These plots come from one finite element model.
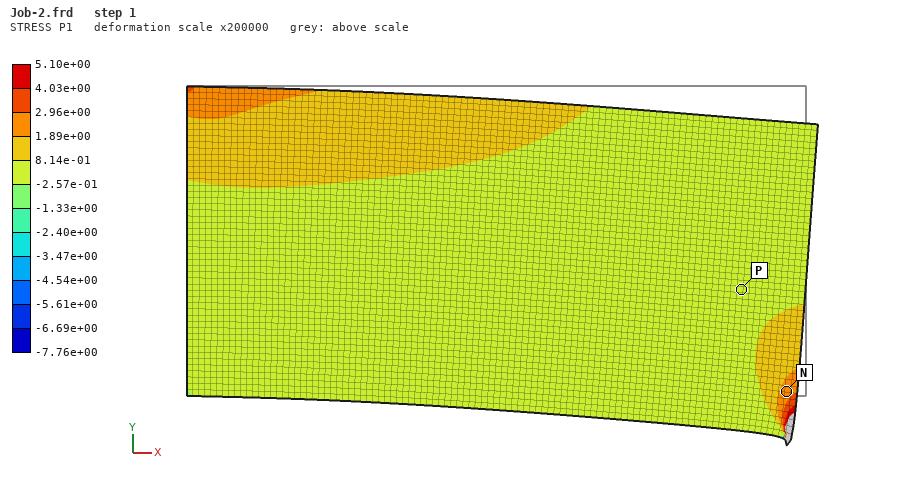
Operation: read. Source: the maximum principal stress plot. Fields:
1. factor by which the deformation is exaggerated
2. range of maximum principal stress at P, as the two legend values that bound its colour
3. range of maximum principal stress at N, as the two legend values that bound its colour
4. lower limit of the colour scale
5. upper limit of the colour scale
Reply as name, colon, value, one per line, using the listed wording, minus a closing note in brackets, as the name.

factor by which the deformation is exaggerated: 200000
range of maximum principal stress at P, as the two legend values that bound its colour: -2.57e-01 to 8.14e-01
range of maximum principal stress at N, as the two legend values that bound its colour: 1.89e+00 to 2.96e+00
lower limit of the colour scale: -7.76e+00
upper limit of the colour scale: 5.10e+00
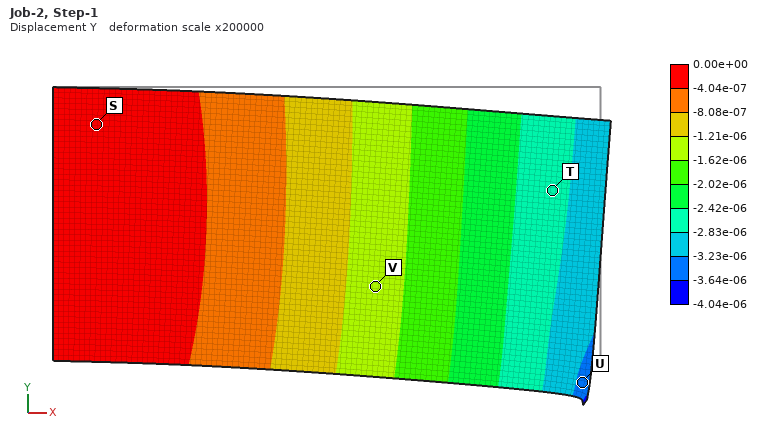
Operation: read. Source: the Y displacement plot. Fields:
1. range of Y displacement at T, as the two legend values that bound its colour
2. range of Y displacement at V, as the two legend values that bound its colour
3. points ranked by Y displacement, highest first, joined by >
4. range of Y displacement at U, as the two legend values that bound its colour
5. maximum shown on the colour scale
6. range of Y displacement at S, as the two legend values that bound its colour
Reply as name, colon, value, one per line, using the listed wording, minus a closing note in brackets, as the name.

range of Y displacement at T, as the two legend values that bound its colour: -2.83e-06 to -2.42e-06
range of Y displacement at V, as the two legend values that bound its colour: -1.62e-06 to -1.21e-06
points ranked by Y displacement, highest first, joined by >: S > V > T > U
range of Y displacement at U, as the two legend values that bound its colour: -3.64e-06 to -3.23e-06
maximum shown on the colour scale: 0.00e+00
range of Y displacement at S, as the two legend values that bound its colour: -4.04e-07 to 0.00e+00
